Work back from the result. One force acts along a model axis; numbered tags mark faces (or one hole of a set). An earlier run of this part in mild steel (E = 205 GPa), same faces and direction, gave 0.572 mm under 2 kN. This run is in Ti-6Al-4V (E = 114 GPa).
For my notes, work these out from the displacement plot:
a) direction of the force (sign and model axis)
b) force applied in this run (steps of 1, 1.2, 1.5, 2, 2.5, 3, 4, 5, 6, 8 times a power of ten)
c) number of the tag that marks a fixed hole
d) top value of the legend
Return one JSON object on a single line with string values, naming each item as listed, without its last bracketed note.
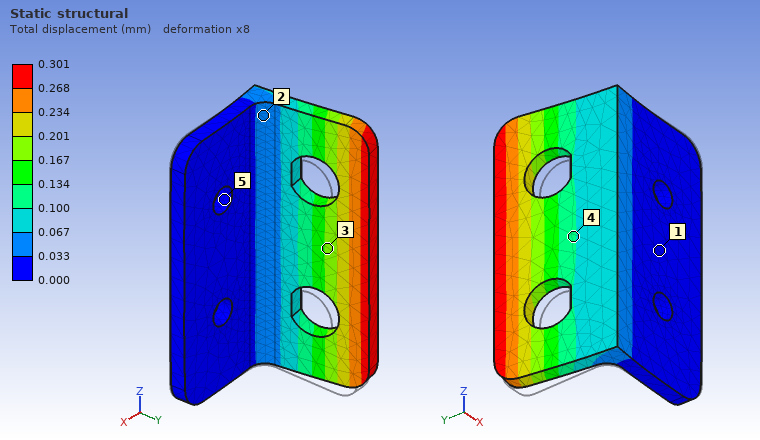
{"direction of the force": "-X", "force applied in this run": "600 N", "number of the tag that marks a fixed hole": "5", "top value of the legend": "0.301 mm"}
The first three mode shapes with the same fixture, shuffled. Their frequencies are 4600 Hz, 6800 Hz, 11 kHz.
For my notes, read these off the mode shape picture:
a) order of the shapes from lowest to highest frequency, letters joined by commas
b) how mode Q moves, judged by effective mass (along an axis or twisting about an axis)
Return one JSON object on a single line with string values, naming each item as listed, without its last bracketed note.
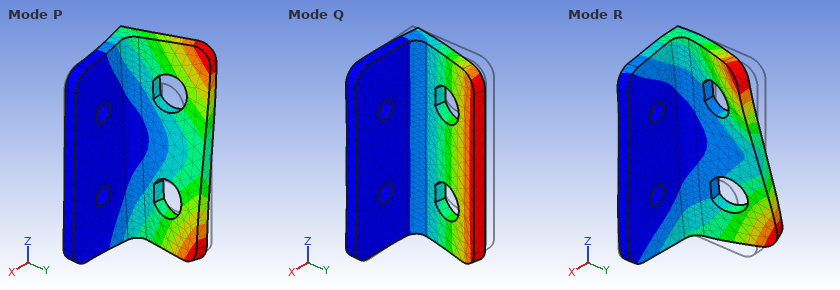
{"order of the shapes from lowest to highest frequency, letters joined by commas": "Q, P, R", "how mode Q moves, judged by effective mass": "along X"}
